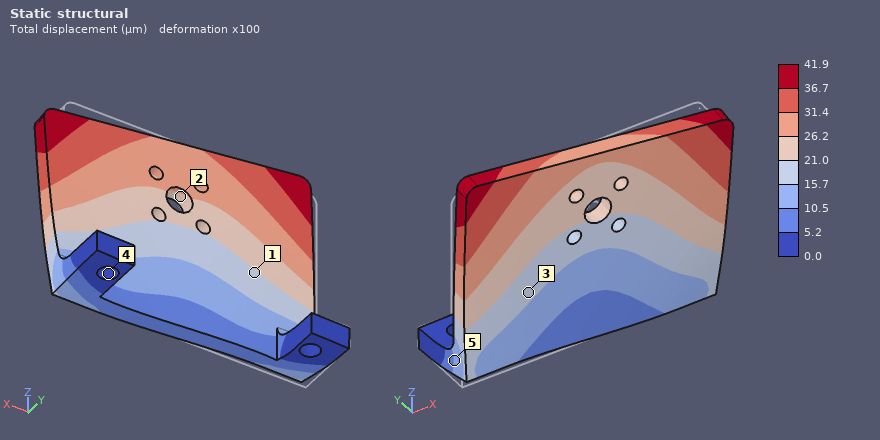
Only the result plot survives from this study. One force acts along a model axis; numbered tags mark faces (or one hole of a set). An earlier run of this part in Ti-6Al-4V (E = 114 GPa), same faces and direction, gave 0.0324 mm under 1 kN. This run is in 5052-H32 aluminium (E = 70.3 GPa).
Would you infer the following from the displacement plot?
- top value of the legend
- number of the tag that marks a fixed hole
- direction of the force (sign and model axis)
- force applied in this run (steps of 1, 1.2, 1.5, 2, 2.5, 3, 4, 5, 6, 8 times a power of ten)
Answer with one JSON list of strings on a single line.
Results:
["41.9 µm", "4", "+X", "800 N"]
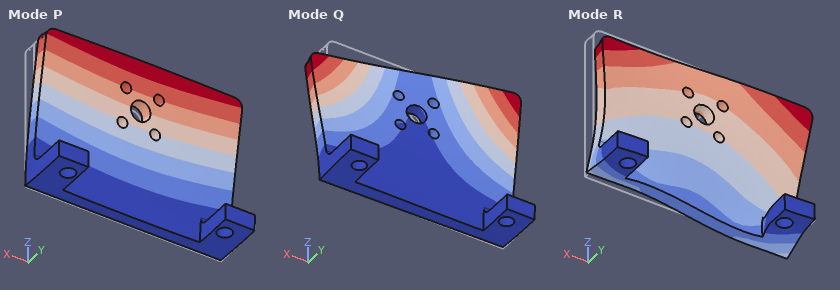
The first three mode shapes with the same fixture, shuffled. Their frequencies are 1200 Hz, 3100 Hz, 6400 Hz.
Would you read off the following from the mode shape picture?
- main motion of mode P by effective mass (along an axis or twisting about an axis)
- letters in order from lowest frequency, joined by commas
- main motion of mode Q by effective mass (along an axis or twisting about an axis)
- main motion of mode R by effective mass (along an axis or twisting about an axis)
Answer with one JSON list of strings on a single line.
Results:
["along Y", "P, Q, R", "twisting about Z", "along X"]
